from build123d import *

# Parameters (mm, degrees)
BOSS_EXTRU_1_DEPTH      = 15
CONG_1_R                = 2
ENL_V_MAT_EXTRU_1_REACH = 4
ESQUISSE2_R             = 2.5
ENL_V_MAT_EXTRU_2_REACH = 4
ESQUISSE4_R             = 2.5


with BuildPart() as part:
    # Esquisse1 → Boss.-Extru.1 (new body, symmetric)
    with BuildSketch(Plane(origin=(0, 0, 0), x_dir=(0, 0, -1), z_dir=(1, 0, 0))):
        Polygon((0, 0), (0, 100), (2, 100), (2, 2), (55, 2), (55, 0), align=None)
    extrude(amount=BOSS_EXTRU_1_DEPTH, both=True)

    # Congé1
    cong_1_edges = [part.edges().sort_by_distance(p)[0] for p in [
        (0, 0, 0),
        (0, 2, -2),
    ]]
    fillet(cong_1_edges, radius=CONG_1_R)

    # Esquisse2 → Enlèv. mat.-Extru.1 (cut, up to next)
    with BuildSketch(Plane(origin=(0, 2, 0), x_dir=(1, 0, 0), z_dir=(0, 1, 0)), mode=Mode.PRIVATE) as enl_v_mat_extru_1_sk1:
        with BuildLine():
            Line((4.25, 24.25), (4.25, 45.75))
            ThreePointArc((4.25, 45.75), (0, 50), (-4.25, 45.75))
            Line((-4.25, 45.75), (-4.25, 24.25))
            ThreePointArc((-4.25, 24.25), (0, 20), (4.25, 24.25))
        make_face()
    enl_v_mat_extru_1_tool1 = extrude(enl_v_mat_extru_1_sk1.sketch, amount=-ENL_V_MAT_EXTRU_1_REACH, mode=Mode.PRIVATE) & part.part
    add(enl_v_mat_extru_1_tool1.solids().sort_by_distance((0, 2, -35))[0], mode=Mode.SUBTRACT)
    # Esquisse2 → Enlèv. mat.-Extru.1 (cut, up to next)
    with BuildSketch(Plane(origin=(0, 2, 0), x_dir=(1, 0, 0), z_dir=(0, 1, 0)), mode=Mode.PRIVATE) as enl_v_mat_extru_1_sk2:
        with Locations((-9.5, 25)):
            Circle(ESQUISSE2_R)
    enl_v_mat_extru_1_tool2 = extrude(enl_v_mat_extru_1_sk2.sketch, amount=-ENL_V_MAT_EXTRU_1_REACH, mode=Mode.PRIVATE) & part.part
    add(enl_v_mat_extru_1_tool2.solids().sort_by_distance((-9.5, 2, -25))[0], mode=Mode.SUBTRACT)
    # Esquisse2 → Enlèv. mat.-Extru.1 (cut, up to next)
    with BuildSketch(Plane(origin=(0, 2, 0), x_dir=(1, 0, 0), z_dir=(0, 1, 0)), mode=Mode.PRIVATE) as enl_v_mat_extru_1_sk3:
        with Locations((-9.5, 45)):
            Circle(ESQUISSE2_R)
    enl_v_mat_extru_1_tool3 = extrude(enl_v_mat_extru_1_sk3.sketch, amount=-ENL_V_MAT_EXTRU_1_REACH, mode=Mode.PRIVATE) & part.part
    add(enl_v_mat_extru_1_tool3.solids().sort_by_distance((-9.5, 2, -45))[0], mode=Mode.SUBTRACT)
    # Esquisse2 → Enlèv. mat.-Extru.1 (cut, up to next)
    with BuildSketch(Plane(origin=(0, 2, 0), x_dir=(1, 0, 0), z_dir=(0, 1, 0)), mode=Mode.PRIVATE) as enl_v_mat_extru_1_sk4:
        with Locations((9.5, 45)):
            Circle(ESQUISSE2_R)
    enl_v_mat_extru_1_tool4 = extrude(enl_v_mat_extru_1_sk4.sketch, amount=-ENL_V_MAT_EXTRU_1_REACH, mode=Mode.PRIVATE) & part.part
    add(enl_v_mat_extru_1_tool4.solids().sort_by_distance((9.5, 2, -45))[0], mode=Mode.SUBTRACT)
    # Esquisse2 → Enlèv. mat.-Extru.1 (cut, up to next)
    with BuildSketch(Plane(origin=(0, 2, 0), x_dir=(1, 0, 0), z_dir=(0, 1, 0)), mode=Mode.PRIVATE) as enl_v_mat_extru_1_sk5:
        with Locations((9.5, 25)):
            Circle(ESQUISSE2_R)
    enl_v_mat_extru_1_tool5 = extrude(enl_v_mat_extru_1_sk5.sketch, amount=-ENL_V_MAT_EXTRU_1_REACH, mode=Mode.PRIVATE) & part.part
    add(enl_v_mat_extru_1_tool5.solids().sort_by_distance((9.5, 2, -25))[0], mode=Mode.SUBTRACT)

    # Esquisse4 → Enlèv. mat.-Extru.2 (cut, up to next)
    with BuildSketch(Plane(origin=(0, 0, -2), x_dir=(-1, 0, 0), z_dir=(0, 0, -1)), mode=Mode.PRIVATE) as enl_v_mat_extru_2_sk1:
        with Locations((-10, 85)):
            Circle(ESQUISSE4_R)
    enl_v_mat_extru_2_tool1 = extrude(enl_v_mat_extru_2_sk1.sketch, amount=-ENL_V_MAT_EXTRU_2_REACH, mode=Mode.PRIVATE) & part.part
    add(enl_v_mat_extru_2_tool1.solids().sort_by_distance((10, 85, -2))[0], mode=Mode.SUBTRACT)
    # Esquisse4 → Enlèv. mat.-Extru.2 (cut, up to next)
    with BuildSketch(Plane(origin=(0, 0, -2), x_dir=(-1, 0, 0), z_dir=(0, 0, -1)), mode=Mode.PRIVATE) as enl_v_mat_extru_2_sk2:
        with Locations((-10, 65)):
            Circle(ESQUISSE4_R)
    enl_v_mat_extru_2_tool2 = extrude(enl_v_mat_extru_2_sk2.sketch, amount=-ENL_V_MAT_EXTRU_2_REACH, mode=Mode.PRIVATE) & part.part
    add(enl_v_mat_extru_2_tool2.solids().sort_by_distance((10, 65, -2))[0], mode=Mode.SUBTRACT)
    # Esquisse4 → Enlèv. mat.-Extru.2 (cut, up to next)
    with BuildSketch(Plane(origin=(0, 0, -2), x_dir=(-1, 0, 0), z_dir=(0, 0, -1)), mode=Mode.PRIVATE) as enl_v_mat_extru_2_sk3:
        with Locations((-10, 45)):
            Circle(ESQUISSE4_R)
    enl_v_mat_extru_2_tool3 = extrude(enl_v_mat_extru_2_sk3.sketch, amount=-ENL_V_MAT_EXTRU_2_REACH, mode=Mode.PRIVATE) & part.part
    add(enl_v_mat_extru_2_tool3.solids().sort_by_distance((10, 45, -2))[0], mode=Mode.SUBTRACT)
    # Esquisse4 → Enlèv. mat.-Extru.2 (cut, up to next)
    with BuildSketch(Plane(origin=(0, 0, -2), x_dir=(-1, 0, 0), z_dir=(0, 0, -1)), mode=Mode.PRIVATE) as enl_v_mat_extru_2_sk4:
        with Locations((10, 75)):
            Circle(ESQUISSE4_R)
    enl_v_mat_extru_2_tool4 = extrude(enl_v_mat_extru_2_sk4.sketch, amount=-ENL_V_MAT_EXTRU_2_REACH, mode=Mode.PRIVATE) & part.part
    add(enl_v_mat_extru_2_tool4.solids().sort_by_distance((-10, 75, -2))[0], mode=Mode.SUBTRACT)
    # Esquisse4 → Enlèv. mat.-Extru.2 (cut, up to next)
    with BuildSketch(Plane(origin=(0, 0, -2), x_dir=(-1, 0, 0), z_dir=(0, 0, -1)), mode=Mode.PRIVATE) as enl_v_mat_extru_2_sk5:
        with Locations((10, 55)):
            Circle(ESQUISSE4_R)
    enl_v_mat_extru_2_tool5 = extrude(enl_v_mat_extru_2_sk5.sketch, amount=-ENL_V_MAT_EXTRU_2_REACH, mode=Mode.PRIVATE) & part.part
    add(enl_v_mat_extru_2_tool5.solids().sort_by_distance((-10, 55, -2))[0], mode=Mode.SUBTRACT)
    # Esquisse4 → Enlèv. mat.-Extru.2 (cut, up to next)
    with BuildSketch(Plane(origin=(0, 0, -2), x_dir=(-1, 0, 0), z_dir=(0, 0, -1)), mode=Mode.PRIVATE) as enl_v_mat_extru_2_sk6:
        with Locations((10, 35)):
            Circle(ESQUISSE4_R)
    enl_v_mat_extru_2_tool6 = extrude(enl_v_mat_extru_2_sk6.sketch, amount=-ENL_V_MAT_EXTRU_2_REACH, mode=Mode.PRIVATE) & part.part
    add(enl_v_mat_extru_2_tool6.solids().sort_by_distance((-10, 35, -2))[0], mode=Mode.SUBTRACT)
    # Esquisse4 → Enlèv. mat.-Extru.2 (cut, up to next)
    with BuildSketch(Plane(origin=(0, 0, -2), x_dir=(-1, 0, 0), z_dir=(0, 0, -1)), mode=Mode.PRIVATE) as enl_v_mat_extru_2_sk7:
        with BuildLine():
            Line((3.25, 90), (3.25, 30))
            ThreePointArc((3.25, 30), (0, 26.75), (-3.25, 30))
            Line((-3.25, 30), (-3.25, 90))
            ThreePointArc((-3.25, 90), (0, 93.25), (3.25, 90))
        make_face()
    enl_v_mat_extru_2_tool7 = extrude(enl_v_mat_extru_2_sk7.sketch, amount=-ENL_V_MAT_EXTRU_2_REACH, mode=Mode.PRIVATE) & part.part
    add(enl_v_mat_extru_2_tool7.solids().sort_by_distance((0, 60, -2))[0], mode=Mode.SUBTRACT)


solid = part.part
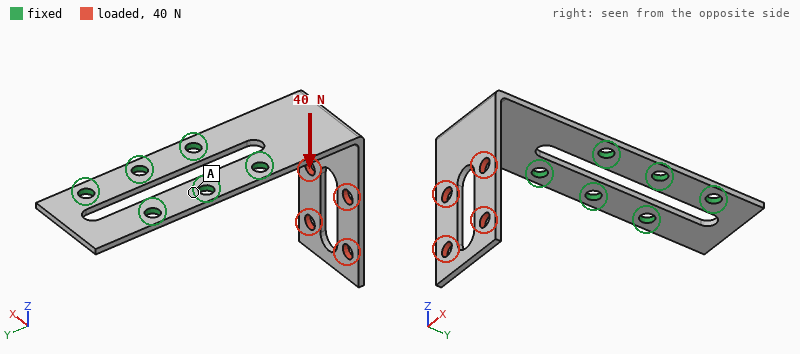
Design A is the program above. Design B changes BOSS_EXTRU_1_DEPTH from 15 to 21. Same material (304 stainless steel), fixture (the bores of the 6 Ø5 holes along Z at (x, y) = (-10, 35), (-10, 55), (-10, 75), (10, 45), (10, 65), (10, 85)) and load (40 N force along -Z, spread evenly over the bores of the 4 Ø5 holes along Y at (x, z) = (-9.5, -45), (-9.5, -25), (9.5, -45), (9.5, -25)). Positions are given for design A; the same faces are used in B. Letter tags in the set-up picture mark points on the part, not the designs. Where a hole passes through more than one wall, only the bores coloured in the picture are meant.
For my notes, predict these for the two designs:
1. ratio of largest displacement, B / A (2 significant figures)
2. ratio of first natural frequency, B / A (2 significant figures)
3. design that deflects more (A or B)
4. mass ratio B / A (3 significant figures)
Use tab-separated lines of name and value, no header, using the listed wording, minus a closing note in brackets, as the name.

ratio of largest displacement, B / A	0.71
ratio of first natural frequency, B / A	0.97
design that deflects more	A
mass ratio B / A	1.49
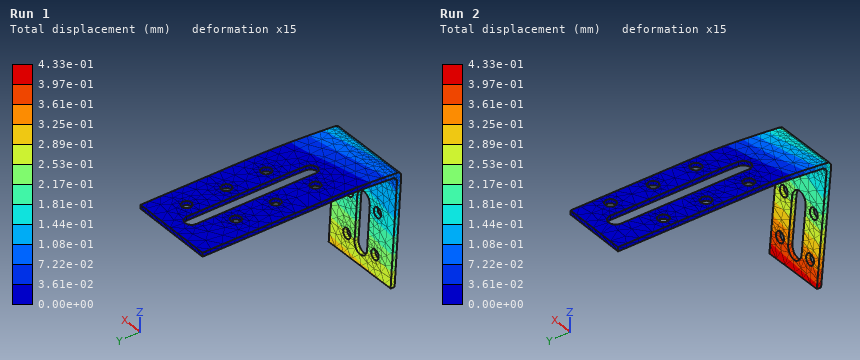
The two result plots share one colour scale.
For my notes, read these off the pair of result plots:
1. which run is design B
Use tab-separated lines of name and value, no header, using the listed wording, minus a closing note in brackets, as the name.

which run is design B	Run 1
